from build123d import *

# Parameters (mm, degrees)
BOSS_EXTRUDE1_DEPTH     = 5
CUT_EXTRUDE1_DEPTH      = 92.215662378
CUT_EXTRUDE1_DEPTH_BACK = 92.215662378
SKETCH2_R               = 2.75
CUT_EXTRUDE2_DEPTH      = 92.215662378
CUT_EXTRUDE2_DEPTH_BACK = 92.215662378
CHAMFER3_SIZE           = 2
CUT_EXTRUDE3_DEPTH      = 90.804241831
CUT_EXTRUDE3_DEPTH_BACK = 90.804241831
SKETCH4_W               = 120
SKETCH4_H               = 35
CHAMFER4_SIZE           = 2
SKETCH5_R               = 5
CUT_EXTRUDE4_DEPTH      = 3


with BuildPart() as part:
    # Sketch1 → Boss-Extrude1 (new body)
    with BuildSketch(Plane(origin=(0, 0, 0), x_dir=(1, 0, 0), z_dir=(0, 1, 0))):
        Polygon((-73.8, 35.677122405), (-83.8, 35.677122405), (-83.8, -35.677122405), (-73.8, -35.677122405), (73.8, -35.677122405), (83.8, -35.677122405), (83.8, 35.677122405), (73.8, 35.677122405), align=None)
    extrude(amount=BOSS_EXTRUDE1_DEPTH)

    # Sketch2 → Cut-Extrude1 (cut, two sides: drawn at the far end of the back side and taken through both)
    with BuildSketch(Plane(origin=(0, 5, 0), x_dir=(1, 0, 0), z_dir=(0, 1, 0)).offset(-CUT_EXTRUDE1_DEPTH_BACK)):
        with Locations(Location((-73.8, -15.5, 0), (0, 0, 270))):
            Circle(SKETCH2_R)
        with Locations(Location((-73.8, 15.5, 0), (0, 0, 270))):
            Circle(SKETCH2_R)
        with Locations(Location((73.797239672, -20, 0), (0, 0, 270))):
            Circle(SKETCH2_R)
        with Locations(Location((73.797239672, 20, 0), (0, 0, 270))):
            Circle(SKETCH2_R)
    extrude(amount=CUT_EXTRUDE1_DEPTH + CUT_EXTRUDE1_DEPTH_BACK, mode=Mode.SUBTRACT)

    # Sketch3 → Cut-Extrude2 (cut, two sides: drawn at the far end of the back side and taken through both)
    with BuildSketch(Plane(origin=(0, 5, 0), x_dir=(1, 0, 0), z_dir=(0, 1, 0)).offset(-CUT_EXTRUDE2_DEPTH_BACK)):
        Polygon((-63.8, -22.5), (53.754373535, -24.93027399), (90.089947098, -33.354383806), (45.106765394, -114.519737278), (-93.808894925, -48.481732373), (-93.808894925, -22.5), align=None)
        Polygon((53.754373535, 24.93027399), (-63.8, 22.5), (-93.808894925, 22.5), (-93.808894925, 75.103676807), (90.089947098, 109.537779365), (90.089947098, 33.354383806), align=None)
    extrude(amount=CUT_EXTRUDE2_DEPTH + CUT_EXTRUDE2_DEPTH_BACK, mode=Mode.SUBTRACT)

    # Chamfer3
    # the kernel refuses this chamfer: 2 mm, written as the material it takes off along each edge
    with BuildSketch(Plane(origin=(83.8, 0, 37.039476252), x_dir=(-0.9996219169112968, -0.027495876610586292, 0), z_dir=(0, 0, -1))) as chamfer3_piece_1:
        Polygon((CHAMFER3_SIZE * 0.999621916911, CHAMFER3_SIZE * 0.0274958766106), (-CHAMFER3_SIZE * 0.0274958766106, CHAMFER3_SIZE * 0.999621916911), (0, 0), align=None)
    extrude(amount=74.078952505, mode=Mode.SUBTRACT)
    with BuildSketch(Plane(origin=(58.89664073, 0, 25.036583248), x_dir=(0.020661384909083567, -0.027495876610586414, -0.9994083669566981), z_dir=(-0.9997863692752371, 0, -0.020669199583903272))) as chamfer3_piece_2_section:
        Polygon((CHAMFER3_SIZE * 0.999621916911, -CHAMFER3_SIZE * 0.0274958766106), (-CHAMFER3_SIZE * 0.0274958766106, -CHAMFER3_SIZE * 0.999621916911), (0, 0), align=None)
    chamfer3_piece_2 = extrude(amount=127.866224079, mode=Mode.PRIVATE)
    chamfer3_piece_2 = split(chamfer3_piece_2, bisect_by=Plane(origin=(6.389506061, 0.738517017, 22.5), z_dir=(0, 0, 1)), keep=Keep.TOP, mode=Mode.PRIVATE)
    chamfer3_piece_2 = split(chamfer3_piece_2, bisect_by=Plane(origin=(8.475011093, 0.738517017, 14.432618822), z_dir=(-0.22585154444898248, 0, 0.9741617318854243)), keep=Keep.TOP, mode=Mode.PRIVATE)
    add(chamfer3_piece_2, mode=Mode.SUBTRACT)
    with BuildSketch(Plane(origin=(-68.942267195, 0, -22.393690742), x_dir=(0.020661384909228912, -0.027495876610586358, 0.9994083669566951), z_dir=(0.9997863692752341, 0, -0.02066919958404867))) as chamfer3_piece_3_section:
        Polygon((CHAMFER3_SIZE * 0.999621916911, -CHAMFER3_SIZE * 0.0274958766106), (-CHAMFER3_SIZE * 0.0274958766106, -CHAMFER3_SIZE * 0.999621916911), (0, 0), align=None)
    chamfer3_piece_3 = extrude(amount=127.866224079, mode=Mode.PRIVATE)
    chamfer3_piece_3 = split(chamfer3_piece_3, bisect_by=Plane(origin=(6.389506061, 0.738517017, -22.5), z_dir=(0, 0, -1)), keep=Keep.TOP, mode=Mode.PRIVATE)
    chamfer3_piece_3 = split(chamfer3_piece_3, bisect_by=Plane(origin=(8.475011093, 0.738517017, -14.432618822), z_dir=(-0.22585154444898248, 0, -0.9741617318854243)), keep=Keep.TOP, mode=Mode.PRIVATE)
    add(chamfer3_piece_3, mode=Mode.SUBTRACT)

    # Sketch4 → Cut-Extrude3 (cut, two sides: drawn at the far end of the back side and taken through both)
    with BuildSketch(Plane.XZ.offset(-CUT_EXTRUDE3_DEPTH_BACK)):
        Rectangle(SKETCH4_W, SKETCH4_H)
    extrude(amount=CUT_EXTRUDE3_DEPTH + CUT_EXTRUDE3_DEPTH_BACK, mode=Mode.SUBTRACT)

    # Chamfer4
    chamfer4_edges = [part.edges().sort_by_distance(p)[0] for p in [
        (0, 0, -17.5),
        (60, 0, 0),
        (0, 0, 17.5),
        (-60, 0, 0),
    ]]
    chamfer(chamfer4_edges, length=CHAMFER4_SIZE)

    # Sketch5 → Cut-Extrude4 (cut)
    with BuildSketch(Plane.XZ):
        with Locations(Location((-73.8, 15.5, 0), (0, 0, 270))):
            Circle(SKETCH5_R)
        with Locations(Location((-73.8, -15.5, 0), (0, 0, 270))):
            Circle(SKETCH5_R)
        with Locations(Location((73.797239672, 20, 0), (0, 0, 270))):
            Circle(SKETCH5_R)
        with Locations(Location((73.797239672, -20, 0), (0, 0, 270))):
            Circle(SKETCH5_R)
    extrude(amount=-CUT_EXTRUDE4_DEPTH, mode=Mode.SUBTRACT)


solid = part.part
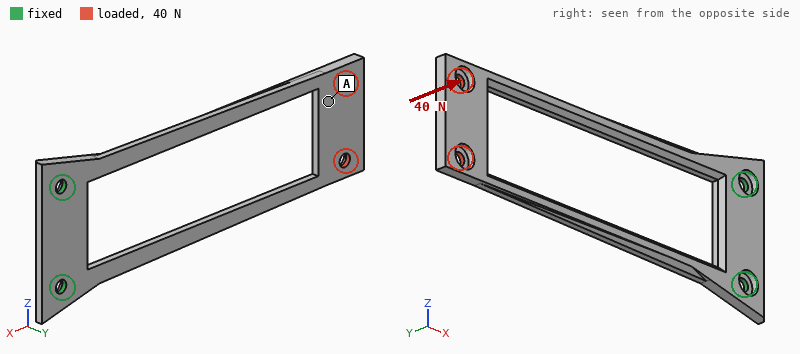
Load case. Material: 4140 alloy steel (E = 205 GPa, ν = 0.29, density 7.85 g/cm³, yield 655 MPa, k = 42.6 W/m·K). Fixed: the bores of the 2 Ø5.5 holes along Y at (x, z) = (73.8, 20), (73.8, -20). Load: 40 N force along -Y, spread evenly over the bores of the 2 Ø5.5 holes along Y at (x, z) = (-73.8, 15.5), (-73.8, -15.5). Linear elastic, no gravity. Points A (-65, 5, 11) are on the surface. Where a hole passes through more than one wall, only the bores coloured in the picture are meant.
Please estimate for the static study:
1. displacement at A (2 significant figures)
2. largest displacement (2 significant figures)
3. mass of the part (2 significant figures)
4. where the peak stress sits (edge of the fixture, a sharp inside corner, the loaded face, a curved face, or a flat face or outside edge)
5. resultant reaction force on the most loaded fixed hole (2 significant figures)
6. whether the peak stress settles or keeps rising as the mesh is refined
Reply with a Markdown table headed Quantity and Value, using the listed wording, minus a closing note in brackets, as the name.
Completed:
| Quantity | Value |
|---|---|
| displacement at A | 1.5 mm |
| largest displacement | 1.8 mm |
| mass of the part | 140 g |
| where the peak stress sits | edge of the fixture |
| resultant reaction force on the most loaded fixed hole | 28 N |
| whether the peak stress settles or keeps rising as the mesh is refined | keeps rising |
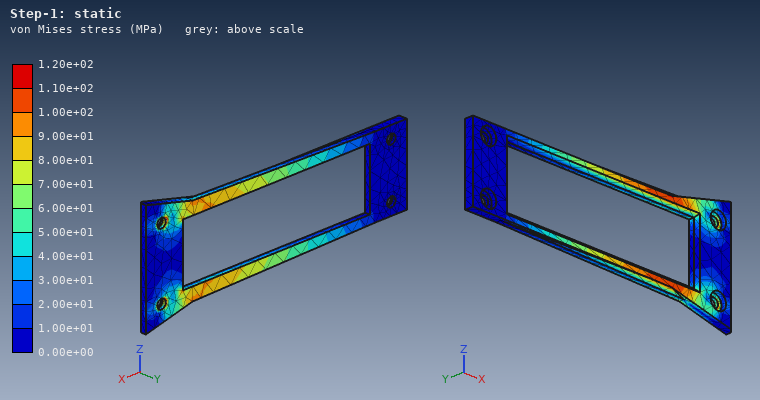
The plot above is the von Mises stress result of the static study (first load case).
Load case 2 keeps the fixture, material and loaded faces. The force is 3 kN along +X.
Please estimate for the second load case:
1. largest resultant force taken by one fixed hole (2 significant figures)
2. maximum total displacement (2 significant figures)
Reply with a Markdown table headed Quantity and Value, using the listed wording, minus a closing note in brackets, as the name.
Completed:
| Quantity | Value |
|---|---|
| largest resultant force taken by one fixed hole | 1.5 kN |
| maximum total displacement | 1.9 mm |
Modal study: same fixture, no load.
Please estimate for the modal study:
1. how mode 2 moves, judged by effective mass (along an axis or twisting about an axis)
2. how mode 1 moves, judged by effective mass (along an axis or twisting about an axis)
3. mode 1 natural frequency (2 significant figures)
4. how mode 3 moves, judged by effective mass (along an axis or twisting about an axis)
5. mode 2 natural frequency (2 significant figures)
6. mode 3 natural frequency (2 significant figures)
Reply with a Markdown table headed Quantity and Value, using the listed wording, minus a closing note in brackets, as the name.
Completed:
| Quantity | Value |
|---|---|
| how mode 2 moves, judged by effective mass | along Z |
| how mode 1 moves, judged by effective mass | along Y |
| mode 1 natural frequency | 120 Hz |
| how mode 3 moves, judged by effective mass | twisting about X |
| mode 2 natural frequency | 320 Hz |
| mode 3 natural frequency | 580 Hz |
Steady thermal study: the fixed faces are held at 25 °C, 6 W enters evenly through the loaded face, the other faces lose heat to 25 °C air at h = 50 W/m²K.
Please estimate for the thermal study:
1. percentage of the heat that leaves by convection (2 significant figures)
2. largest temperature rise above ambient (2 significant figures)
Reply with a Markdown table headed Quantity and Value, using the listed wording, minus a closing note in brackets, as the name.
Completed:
| Quantity | Value |
|---|---|
| percentage of the heat that leaves by convection | 99 % |
| largest temperature rise above ambient | 37 K |
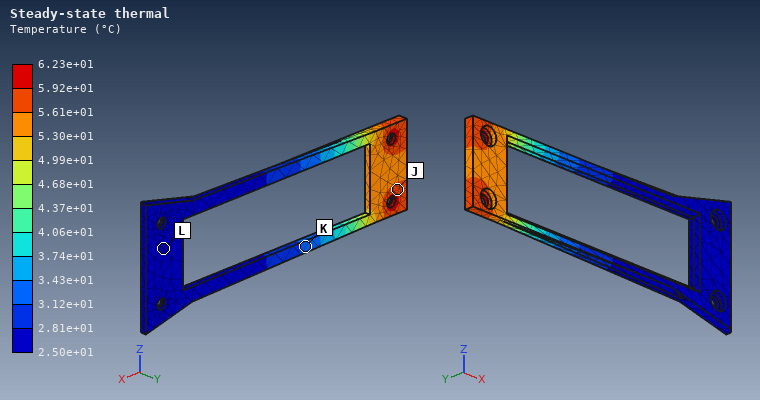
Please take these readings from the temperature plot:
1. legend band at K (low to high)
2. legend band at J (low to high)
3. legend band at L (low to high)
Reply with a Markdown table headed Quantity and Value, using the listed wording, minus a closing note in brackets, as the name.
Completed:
| Quantity | Value |
|---|---|
| legend band at K | 3.12e+01 to 3.43e+01 °C |
| legend band at J | 5.61e+01 to 5.92e+01 °C |
| legend band at L | 2.50e+01 to 2.81e+01 °C |
